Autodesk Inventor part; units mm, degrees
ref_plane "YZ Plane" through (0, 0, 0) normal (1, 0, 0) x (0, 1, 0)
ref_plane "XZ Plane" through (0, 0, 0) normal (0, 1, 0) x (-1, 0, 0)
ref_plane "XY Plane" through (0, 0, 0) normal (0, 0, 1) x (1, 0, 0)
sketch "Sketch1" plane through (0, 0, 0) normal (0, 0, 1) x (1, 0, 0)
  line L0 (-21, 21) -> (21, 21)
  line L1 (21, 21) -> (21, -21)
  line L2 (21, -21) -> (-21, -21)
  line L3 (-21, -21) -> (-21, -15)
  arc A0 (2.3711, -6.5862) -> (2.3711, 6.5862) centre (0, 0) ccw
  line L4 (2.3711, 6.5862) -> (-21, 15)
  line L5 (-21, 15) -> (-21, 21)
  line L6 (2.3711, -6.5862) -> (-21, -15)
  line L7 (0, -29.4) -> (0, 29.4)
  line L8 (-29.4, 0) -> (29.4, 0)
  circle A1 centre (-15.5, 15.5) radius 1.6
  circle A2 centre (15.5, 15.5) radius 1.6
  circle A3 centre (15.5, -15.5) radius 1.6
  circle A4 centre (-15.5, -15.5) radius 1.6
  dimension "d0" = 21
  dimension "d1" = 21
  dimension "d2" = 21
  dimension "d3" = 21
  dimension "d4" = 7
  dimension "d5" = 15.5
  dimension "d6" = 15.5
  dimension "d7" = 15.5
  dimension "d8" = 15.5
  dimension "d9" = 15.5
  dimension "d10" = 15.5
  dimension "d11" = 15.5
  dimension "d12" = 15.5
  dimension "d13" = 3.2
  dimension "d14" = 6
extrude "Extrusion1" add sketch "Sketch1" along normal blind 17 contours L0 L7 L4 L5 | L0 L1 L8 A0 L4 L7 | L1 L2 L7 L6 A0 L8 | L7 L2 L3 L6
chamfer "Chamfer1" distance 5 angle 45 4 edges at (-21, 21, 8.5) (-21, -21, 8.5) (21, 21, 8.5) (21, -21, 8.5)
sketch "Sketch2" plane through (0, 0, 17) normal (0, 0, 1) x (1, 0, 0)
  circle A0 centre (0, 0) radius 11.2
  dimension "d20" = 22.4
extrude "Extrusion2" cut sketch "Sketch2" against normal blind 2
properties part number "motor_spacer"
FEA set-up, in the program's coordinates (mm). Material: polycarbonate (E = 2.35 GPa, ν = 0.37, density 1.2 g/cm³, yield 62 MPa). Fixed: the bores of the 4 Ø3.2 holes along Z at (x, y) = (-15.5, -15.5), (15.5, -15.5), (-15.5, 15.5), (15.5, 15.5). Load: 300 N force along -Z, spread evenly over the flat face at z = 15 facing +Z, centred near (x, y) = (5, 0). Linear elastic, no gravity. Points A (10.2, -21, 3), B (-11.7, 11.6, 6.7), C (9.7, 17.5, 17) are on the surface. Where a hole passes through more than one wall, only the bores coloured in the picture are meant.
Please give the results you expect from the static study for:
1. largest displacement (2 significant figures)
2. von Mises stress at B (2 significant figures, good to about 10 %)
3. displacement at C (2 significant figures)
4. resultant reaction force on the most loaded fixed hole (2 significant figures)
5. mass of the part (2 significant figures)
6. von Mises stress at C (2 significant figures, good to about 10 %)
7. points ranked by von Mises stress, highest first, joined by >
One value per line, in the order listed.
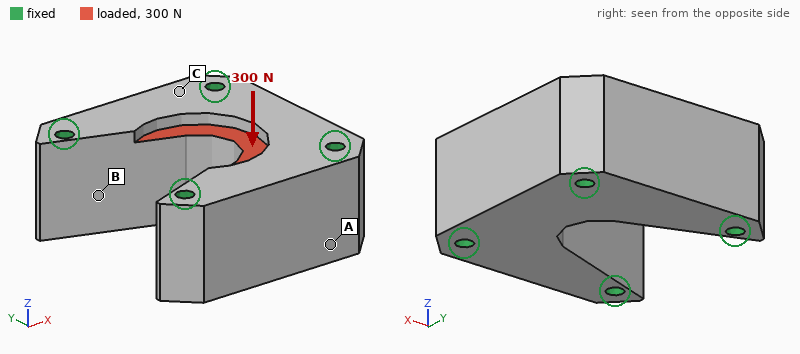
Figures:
18 µm
1.3 MPa
4.2 µm
100 N
23 g
0.55 MPa
B > C > A
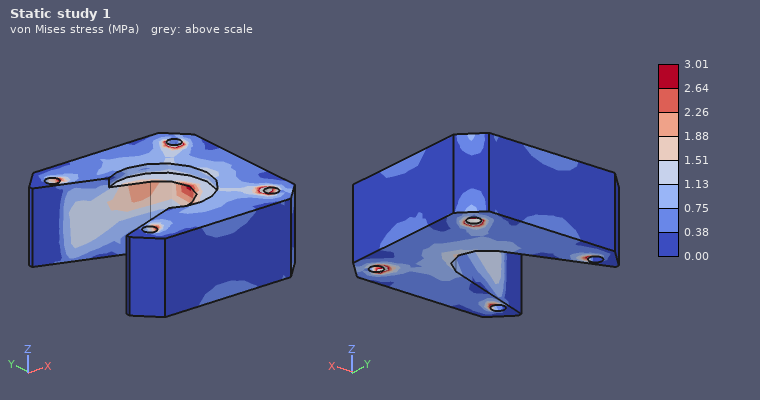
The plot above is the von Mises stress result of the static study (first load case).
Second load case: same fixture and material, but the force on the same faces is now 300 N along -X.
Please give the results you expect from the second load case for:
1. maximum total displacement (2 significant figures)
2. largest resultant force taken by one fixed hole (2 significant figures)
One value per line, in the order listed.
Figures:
19 µm
110 N
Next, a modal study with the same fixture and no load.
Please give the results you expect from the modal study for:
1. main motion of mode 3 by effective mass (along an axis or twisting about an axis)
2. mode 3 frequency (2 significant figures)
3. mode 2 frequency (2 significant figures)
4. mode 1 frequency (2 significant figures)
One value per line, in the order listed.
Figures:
along Y
10 kHz
9300 Hz
9000 Hz
